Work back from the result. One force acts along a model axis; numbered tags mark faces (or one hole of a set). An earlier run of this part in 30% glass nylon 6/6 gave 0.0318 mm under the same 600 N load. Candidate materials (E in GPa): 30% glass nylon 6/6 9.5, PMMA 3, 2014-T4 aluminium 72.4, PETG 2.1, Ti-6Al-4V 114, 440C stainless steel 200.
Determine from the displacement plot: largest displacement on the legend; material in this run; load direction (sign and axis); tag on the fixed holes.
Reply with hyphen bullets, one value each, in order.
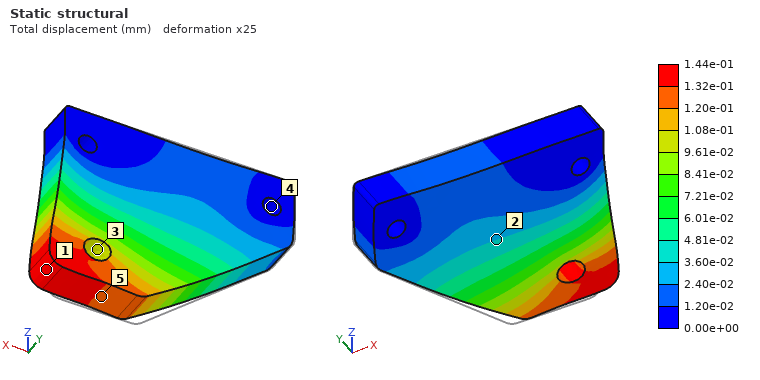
- 1.44e-01 mm
- PETG
- +X
- 4
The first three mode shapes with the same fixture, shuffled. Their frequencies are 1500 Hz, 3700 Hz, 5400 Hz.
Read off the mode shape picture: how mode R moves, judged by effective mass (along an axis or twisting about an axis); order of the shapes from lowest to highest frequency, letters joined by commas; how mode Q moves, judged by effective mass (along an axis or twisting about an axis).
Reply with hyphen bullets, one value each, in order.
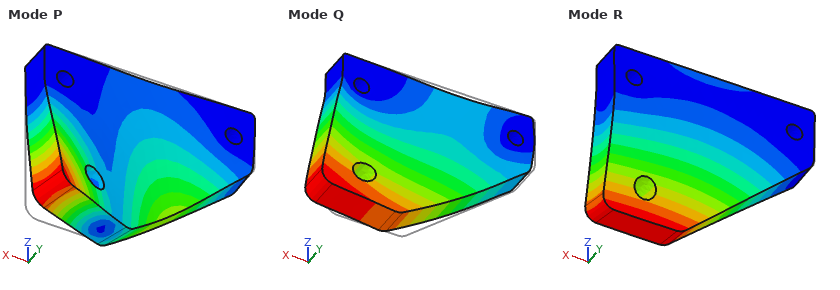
- along Y
- R, P, Q
- along X
